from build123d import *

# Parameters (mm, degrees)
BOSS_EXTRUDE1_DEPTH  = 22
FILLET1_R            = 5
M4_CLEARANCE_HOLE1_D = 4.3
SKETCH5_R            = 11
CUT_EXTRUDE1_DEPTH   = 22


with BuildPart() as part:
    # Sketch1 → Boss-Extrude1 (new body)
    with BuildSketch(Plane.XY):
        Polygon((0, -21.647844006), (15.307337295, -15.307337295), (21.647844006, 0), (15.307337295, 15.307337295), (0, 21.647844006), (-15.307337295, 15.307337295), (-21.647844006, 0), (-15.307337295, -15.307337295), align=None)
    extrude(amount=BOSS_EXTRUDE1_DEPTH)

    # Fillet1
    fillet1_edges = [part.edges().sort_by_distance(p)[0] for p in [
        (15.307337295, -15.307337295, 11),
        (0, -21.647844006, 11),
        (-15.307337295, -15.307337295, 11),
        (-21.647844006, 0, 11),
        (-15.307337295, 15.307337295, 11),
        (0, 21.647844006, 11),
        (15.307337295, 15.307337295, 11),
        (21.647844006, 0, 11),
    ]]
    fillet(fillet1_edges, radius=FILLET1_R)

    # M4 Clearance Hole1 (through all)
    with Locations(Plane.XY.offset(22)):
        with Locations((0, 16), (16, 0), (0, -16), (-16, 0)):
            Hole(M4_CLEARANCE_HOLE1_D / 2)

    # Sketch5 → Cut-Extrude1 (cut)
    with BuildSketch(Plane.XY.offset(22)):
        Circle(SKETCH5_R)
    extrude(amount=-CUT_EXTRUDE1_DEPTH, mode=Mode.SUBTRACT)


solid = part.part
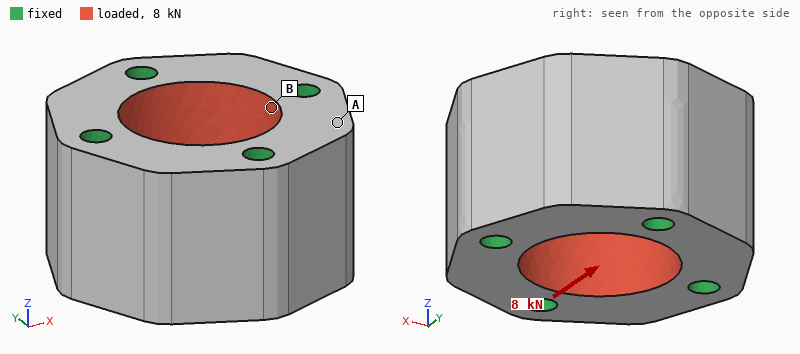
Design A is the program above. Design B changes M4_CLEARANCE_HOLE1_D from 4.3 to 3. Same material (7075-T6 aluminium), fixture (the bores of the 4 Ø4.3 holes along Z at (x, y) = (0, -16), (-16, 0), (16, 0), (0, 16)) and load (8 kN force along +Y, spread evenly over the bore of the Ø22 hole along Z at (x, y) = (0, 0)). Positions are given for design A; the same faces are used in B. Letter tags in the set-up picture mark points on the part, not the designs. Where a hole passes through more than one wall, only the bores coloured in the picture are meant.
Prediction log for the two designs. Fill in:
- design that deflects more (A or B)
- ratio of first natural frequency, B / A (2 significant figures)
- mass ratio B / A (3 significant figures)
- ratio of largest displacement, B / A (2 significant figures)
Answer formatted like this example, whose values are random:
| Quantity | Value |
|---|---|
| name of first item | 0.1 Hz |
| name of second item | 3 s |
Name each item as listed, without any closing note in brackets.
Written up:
| Quantity | Value |
|---|---|
| design that deflects more | B |
| ratio of first natural frequency, B / A | 0.90 |
| mass ratio B / A | 1.03 |
| ratio of largest displacement, B / A | 1.1 |
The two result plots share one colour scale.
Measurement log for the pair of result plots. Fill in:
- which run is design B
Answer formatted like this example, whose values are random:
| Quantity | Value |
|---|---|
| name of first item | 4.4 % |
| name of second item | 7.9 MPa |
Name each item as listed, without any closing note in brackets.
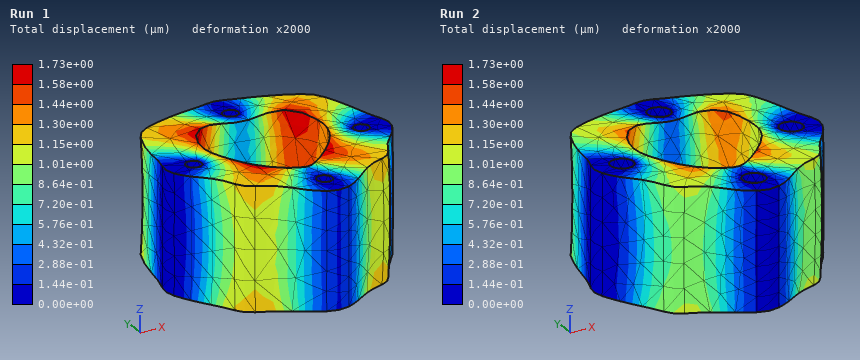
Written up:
| Quantity | Value |
|---|---|
| which run is design B | Run 1 |
